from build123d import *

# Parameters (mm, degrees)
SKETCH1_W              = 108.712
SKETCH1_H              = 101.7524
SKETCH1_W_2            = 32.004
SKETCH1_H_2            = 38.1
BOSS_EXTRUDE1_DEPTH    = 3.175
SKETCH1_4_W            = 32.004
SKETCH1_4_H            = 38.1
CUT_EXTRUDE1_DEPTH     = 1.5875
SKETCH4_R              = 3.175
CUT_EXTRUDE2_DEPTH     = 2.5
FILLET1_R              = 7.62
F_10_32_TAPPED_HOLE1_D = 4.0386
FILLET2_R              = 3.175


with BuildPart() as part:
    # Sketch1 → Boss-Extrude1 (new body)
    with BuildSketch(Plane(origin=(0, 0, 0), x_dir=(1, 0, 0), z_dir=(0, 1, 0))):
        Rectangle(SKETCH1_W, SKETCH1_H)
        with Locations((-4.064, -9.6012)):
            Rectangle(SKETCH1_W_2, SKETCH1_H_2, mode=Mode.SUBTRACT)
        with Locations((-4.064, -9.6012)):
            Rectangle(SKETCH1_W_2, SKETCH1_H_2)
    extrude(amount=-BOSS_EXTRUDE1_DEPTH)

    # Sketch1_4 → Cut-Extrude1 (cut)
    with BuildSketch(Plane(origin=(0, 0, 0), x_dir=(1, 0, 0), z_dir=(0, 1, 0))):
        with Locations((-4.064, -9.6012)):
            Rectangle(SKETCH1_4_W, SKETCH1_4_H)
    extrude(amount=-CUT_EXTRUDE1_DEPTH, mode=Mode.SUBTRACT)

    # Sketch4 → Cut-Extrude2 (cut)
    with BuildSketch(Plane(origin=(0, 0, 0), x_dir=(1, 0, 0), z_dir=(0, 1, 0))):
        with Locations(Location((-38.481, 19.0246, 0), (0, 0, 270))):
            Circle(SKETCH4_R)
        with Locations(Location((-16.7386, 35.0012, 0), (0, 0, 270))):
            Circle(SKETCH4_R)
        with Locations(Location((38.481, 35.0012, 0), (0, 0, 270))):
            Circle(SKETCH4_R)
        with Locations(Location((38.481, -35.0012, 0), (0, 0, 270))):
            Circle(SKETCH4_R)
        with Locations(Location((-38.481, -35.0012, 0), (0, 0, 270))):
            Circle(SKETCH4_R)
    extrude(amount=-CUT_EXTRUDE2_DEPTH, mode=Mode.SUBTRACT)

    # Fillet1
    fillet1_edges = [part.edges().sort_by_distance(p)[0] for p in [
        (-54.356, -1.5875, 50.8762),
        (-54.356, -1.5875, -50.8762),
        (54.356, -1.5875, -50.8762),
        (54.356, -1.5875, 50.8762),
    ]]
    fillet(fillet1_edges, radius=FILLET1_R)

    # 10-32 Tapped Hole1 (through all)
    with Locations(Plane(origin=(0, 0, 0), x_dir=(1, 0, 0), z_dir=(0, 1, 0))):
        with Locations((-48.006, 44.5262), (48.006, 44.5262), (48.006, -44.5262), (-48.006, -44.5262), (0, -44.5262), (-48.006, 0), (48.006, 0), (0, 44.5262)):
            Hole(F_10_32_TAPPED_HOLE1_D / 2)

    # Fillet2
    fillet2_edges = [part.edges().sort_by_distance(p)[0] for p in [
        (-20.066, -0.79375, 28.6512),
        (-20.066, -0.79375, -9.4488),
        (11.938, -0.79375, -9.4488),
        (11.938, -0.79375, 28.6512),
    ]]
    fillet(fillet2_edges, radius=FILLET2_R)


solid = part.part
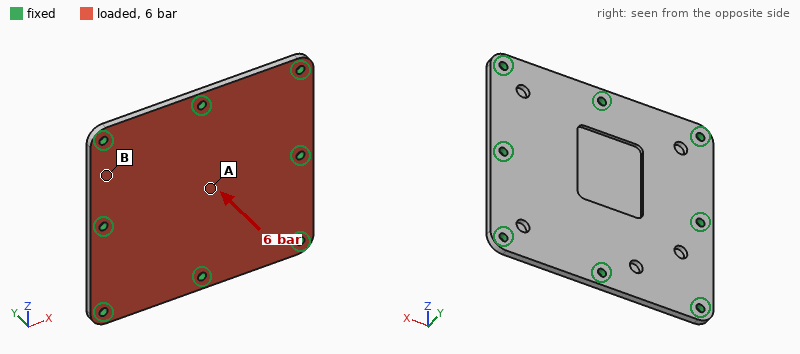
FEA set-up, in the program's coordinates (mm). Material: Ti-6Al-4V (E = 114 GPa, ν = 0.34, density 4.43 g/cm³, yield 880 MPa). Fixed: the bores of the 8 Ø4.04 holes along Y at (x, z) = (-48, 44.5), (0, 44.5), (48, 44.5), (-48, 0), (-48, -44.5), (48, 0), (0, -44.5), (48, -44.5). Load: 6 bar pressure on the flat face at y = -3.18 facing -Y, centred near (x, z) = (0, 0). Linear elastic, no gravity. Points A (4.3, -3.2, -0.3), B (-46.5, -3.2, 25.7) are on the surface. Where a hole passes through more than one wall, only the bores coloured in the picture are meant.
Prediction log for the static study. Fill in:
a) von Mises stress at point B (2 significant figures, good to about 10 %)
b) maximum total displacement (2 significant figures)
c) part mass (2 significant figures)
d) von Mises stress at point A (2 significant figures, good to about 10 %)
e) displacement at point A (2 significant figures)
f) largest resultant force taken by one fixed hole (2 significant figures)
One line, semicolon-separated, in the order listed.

40 MPa; 0.32 mm; 140 g; 120 MPa; 0.30 mm; 1.4 kN
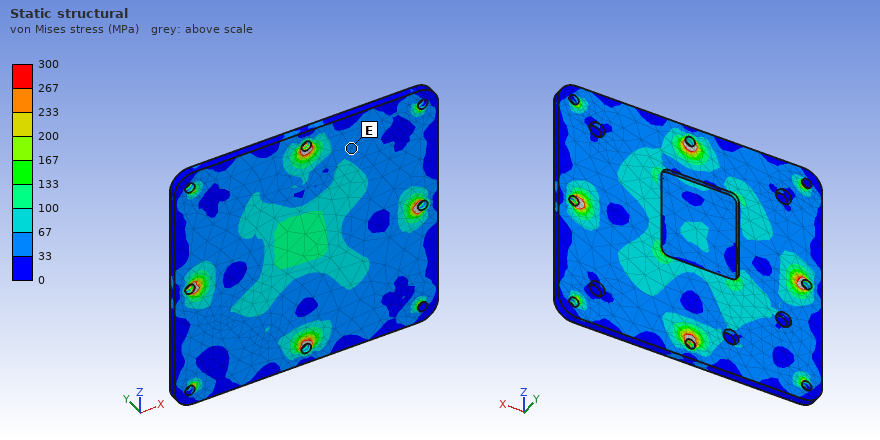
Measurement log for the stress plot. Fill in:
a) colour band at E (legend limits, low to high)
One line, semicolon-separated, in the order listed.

33 to 67 MPa
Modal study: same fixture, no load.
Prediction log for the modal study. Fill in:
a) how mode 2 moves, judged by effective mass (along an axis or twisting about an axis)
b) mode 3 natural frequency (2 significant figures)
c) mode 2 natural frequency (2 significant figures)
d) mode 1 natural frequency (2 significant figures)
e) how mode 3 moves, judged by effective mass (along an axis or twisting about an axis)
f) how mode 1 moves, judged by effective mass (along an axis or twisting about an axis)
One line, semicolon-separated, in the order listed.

twisting about Z; 5000 Hz; 4500 Hz; 2800 Hz; twisting about X; along Y
